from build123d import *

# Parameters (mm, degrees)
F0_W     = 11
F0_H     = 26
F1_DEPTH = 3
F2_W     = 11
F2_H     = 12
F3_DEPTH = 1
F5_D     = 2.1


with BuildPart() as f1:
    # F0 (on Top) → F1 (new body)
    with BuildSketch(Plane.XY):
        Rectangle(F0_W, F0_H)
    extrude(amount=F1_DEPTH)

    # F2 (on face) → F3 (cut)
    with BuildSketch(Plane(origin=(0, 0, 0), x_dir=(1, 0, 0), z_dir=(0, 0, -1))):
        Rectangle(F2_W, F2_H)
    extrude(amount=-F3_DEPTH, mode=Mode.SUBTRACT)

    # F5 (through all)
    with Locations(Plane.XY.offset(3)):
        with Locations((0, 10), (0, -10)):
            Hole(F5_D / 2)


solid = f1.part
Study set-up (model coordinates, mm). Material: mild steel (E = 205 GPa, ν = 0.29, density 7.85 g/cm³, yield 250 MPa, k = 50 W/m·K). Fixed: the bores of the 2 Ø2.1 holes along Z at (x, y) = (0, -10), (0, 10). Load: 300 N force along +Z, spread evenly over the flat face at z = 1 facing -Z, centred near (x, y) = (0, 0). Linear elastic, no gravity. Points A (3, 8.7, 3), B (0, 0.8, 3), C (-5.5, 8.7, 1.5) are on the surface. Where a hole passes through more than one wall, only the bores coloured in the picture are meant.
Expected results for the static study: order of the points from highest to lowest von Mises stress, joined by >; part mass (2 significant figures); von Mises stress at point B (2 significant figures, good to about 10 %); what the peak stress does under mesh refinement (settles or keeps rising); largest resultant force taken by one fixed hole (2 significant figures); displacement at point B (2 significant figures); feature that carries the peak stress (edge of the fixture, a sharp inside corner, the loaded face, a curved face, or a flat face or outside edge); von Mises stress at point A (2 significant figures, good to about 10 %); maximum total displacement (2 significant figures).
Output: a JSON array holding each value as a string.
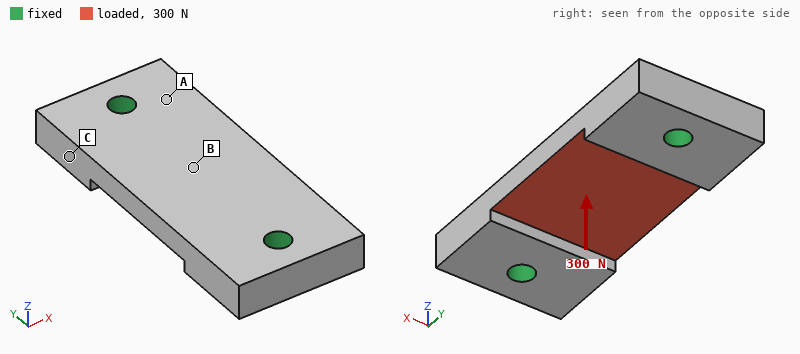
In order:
["B > A > C", "5.5 g", "37 MPa", "keeps rising", "170 N", "3.8 µm", "edge of the fixture", "19 MPa", "4.4 µm"]
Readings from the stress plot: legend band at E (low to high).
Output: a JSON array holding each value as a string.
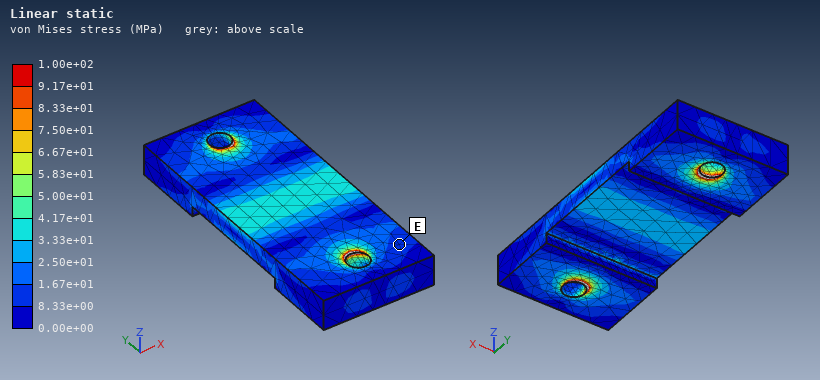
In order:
["8.33e+00 to 1.67e+01 MPa"]
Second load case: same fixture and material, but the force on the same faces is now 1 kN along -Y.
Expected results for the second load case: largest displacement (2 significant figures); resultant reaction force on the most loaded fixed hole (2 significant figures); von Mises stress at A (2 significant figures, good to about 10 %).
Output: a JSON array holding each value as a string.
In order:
["1.2 µm", "500 N", "20 MPa"]
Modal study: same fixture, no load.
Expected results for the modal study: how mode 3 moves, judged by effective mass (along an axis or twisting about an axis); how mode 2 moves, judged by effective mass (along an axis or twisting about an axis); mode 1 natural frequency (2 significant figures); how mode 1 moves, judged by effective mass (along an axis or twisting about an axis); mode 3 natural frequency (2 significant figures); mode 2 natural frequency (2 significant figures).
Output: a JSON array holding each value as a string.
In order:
["along X", "twisting about Y", "32 kHz", "along Z", "54 kHz", "38 kHz"]
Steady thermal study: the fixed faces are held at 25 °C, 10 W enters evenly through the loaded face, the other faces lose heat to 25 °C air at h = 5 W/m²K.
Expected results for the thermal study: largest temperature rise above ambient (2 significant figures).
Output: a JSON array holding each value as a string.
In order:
["30 K"]
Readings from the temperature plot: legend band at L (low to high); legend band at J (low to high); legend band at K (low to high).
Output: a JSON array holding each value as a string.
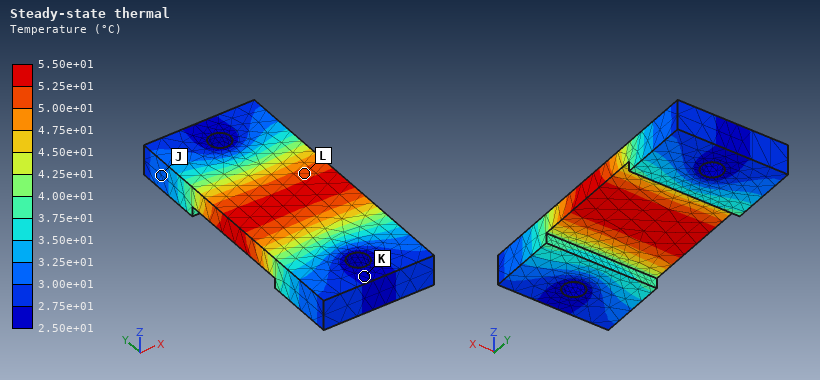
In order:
["5.00e+01 to 5.25e+01 °C", "3.00e+01 to 3.25e+01 °C", "2.50e+01 to 2.75e+01 °C"]
